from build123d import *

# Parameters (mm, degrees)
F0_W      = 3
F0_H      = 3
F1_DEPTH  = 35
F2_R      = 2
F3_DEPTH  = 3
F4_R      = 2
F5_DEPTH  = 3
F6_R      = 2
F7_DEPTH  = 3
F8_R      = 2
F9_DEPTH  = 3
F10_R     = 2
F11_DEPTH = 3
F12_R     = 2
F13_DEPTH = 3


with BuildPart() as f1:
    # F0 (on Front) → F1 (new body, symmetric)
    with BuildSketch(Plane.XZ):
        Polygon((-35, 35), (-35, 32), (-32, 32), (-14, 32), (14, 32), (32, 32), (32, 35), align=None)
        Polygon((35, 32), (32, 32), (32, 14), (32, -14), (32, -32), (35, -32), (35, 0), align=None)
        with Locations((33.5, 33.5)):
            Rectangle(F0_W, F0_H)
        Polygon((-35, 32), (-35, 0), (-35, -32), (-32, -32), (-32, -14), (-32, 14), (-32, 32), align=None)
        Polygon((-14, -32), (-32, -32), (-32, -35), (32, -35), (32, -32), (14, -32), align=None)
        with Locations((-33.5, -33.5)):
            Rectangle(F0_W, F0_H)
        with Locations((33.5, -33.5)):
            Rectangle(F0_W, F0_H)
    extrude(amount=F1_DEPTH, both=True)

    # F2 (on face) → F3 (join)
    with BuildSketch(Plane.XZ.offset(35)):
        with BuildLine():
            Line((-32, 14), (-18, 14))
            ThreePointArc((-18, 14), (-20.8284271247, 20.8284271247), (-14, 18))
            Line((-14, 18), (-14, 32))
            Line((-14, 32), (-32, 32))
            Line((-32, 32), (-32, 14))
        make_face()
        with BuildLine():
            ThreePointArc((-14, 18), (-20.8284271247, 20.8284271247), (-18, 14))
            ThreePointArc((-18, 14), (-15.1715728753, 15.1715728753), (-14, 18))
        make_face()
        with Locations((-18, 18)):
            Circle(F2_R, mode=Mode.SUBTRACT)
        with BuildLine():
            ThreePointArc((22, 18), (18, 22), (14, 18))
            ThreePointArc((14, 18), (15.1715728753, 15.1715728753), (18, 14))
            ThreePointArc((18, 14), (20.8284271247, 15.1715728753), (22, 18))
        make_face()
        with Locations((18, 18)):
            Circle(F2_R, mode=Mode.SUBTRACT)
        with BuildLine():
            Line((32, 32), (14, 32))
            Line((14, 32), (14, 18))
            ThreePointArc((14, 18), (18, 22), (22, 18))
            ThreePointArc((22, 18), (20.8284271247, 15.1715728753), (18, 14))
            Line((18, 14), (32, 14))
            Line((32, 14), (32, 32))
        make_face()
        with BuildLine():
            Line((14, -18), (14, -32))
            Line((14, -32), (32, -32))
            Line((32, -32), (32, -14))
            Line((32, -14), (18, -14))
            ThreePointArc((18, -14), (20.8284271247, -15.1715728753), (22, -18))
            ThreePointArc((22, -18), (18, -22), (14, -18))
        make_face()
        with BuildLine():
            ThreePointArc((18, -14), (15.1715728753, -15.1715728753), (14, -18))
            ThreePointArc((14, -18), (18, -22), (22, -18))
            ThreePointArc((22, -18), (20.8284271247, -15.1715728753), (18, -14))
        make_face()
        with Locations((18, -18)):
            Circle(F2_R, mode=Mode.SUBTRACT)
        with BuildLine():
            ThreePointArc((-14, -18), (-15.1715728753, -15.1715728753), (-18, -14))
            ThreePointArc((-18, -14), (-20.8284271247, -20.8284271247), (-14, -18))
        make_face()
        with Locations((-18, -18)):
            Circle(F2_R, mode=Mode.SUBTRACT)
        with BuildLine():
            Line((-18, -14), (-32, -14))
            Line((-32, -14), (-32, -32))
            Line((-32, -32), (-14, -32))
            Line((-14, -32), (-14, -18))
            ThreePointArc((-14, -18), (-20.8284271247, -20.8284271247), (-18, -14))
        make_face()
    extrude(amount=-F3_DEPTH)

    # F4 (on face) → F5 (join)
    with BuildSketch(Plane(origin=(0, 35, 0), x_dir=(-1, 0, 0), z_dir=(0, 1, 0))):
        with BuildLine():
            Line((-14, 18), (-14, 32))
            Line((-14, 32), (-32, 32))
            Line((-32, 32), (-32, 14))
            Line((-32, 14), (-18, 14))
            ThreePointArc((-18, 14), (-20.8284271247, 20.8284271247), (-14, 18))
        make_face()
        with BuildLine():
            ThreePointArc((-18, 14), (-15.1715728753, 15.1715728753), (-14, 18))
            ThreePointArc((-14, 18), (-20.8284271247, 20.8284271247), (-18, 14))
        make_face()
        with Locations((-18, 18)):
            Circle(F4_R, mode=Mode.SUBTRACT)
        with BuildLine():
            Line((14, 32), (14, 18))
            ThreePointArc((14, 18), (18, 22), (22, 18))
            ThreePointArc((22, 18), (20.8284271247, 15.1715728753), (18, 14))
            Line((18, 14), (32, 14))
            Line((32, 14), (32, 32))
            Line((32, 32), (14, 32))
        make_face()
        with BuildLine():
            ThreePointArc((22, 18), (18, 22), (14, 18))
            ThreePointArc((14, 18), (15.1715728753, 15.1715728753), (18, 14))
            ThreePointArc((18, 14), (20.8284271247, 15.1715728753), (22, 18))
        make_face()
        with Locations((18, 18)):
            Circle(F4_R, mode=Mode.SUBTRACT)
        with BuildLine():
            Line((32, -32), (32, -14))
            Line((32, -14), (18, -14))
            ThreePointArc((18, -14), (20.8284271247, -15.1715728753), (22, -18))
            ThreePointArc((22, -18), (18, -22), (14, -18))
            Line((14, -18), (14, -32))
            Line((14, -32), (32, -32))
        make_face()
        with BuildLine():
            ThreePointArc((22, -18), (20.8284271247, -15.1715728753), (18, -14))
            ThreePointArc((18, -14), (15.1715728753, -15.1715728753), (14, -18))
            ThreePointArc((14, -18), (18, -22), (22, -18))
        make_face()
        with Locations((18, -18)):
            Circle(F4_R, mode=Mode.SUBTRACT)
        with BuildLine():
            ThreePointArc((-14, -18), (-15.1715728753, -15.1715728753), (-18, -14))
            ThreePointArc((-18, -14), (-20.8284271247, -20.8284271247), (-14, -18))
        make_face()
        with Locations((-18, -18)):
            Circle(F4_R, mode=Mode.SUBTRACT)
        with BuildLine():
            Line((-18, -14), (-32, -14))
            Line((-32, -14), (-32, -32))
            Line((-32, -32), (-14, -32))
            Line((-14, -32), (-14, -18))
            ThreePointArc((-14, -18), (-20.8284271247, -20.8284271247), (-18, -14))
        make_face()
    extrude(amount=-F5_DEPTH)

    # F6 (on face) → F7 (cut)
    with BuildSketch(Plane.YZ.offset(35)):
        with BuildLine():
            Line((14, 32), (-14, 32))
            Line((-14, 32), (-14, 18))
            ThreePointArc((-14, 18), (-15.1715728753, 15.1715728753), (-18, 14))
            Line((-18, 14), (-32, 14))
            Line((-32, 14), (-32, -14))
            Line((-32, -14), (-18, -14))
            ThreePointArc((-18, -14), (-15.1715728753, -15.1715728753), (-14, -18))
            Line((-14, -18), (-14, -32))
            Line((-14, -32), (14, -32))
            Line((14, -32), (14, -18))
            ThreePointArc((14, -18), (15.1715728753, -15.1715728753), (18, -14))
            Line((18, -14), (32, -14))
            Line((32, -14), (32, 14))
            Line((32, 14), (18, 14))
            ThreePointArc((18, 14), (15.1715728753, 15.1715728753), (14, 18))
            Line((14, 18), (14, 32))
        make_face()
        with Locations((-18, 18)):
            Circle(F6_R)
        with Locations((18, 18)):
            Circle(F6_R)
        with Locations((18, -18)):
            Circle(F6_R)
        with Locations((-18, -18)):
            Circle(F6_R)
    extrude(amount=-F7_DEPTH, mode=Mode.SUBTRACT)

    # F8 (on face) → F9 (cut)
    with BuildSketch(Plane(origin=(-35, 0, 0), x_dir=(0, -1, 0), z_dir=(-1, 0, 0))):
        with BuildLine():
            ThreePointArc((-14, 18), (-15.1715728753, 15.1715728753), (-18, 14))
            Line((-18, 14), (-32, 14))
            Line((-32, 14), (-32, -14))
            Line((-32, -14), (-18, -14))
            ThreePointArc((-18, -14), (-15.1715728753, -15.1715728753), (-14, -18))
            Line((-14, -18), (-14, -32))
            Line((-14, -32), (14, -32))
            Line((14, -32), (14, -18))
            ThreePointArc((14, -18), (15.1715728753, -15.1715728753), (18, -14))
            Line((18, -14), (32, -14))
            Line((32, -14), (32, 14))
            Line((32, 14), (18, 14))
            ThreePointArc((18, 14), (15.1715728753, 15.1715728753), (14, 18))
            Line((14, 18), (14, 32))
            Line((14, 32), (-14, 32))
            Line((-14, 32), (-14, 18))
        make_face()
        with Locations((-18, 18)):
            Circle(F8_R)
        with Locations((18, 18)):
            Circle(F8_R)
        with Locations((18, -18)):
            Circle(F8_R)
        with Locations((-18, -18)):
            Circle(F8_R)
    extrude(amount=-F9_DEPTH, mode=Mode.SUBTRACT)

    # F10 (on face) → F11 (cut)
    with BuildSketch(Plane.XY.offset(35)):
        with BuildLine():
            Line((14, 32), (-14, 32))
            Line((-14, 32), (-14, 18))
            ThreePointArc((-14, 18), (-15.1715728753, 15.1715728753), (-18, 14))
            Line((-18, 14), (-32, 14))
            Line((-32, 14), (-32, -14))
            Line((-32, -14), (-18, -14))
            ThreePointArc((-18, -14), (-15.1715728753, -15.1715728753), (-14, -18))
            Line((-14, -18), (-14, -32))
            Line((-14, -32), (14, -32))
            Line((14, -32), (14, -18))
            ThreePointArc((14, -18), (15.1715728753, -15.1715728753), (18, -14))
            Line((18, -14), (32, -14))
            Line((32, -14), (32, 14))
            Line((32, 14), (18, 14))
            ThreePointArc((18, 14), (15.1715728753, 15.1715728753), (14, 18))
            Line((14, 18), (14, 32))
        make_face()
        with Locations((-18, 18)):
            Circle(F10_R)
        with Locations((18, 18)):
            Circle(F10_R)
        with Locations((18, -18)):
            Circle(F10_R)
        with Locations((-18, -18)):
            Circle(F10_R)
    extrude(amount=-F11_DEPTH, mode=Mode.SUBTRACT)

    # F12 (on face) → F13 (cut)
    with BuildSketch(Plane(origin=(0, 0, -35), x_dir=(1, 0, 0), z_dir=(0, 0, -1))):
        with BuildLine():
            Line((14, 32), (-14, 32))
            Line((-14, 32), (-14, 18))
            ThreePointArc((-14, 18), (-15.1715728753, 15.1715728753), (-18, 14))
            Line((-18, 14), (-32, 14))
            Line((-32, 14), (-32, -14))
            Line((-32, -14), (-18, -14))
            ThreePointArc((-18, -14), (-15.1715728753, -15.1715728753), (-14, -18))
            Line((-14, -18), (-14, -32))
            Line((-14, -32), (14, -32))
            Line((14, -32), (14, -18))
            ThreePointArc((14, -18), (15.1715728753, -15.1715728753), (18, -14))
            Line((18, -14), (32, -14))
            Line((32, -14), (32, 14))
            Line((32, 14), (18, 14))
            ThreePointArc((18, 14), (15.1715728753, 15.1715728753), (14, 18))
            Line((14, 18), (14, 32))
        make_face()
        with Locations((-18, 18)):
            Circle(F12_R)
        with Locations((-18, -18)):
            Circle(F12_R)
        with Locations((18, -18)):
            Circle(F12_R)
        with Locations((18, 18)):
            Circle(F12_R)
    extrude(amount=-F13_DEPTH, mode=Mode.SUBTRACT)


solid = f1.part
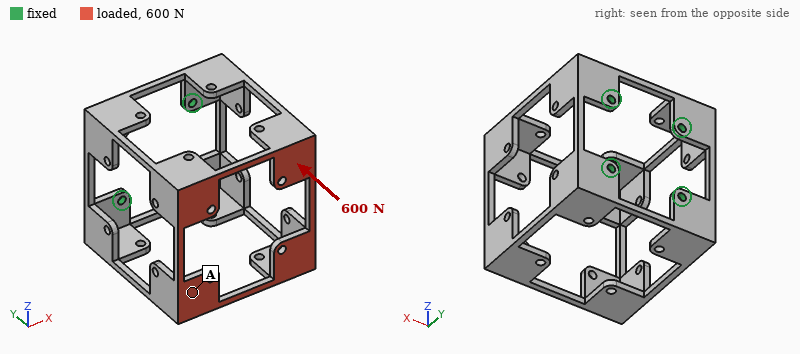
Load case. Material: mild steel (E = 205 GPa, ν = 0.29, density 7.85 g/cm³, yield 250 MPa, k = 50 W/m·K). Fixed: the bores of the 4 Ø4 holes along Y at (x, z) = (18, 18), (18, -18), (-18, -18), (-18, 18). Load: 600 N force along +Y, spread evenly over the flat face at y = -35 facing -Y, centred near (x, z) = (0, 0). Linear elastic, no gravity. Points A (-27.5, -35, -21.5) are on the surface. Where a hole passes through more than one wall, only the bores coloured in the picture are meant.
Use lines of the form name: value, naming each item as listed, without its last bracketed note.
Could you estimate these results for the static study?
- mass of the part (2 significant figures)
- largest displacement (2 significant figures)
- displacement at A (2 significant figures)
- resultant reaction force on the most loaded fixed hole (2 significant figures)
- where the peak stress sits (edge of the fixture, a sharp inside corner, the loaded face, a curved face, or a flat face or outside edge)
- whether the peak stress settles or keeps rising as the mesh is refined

mass of the part: 230 g
largest displacement: 0.22 mm
displacement at A: 0.14 mm
resultant reaction force on the most loaded fixed hole: 150 N
where the peak stress sits: edge of the fixture
whether the peak stress settles or keeps rising as the mesh is refined: keeps rising
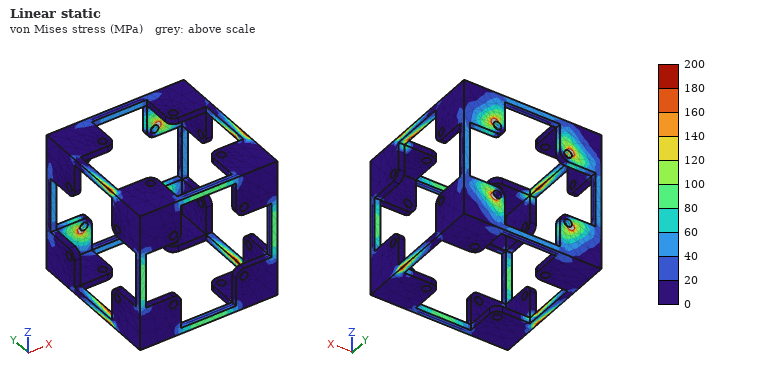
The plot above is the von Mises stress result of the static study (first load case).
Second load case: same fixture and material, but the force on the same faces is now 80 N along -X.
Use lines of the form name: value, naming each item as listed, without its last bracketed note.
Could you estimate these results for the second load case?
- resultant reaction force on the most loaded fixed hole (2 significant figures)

resultant reaction force on the most loaded fixed hole: 40 N
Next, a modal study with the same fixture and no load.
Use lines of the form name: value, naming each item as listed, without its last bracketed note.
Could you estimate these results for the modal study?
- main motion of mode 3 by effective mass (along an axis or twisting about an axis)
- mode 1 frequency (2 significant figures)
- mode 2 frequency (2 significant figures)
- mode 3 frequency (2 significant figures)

main motion of mode 3 by effective mass: twisting about Y
mode 1 frequency: 450 Hz
mode 2 frequency: 450 Hz
mode 3 frequency: 690 Hz
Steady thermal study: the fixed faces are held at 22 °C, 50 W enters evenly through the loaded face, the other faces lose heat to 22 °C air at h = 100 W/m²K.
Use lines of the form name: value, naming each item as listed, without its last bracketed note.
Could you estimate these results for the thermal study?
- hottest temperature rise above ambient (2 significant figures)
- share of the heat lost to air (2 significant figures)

hottest temperature rise above ambient: 61 K
share of the heat lost to air: 99 %
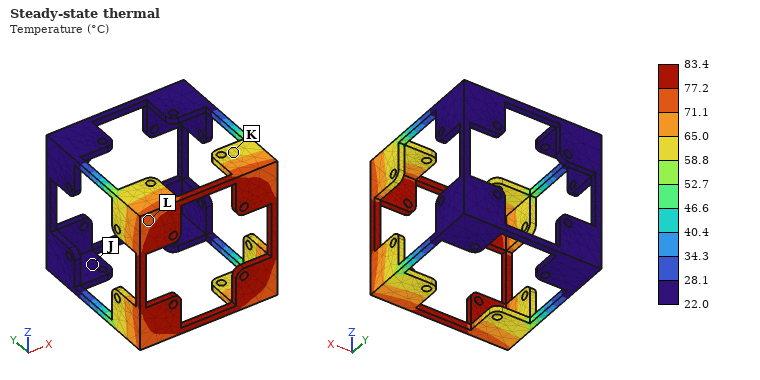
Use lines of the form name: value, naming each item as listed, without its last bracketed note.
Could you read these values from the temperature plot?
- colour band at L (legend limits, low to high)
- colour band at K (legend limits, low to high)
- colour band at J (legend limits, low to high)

colour band at L: 71.1 to 77.2 °C
colour band at K: 58.8 to 65.0 °C
colour band at J: 22.0 to 28.1 °C
